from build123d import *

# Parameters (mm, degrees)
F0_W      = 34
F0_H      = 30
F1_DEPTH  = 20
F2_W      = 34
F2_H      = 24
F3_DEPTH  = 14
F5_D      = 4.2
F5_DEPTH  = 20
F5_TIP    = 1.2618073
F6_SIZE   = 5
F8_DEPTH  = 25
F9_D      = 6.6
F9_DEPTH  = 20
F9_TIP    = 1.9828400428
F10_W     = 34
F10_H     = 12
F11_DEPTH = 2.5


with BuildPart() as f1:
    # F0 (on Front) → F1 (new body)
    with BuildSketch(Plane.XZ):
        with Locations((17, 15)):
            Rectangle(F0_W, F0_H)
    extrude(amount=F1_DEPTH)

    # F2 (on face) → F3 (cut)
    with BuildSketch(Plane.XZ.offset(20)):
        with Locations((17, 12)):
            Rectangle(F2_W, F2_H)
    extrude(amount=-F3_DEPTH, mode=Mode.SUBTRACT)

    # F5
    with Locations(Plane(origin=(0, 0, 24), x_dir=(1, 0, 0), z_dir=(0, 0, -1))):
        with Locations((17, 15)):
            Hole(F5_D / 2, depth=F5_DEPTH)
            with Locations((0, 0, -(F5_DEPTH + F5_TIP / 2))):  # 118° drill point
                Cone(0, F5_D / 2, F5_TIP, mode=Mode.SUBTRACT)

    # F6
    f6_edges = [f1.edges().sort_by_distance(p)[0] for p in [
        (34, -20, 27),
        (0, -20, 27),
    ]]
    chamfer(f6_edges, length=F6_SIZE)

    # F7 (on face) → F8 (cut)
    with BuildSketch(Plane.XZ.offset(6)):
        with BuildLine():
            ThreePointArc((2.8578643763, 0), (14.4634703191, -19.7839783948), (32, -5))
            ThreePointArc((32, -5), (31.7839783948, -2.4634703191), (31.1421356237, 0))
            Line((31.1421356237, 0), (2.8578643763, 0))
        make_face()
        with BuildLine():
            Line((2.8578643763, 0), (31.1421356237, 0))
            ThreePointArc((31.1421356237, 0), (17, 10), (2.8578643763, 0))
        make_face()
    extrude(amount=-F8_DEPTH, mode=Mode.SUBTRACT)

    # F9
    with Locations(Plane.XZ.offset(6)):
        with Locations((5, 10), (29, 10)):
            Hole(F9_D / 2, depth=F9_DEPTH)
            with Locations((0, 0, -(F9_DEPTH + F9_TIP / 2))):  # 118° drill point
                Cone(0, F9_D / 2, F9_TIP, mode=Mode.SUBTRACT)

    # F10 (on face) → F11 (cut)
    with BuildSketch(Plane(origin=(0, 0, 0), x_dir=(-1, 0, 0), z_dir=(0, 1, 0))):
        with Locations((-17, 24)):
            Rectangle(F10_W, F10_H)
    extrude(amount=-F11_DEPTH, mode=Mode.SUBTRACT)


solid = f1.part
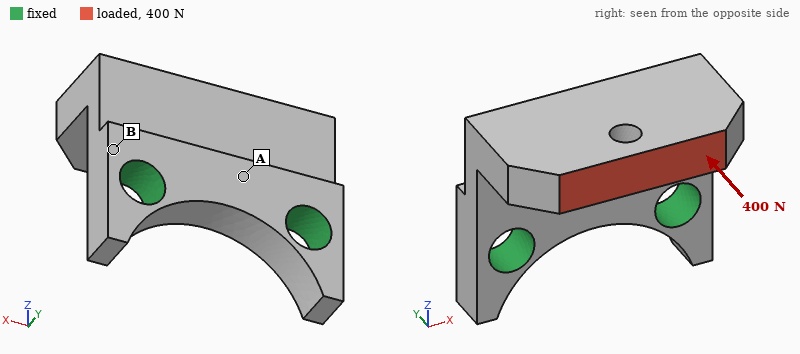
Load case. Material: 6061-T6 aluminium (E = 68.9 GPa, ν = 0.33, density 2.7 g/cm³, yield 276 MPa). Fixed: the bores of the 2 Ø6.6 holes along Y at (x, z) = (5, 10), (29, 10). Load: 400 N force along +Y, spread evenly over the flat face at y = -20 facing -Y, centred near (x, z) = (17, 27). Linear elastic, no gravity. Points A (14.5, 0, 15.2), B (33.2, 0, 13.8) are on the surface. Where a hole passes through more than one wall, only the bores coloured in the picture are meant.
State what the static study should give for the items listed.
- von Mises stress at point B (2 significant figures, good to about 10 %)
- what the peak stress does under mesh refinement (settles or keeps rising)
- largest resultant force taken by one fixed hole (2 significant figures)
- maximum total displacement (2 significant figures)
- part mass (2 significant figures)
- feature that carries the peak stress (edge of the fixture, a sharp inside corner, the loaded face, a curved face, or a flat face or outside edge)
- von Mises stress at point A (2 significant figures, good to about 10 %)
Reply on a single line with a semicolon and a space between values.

20 MPa; keeps rising; 200 N; 62 µm; 16 g; edge of the fixture; 9.0 MPa
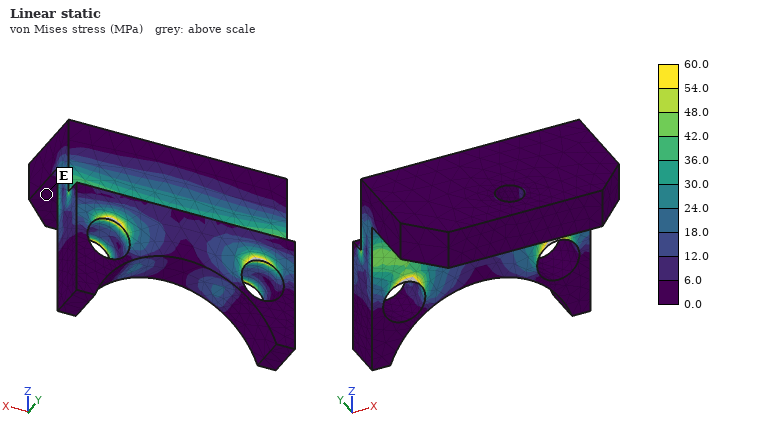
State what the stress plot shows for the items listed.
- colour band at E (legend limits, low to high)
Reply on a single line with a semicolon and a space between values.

0.0 to 6.0 MPa
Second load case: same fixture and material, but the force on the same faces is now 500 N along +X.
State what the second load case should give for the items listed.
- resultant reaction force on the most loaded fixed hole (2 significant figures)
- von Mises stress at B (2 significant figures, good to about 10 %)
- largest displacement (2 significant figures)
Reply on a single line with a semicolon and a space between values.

500 N; 26 MPa; 32 µm
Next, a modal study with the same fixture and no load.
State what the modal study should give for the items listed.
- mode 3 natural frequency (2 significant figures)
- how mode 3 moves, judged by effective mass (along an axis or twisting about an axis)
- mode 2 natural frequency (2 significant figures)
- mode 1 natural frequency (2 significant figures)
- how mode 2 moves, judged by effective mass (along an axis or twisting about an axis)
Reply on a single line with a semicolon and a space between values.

15 kHz; along Y; 9300 Hz; 4400 Hz; along X
